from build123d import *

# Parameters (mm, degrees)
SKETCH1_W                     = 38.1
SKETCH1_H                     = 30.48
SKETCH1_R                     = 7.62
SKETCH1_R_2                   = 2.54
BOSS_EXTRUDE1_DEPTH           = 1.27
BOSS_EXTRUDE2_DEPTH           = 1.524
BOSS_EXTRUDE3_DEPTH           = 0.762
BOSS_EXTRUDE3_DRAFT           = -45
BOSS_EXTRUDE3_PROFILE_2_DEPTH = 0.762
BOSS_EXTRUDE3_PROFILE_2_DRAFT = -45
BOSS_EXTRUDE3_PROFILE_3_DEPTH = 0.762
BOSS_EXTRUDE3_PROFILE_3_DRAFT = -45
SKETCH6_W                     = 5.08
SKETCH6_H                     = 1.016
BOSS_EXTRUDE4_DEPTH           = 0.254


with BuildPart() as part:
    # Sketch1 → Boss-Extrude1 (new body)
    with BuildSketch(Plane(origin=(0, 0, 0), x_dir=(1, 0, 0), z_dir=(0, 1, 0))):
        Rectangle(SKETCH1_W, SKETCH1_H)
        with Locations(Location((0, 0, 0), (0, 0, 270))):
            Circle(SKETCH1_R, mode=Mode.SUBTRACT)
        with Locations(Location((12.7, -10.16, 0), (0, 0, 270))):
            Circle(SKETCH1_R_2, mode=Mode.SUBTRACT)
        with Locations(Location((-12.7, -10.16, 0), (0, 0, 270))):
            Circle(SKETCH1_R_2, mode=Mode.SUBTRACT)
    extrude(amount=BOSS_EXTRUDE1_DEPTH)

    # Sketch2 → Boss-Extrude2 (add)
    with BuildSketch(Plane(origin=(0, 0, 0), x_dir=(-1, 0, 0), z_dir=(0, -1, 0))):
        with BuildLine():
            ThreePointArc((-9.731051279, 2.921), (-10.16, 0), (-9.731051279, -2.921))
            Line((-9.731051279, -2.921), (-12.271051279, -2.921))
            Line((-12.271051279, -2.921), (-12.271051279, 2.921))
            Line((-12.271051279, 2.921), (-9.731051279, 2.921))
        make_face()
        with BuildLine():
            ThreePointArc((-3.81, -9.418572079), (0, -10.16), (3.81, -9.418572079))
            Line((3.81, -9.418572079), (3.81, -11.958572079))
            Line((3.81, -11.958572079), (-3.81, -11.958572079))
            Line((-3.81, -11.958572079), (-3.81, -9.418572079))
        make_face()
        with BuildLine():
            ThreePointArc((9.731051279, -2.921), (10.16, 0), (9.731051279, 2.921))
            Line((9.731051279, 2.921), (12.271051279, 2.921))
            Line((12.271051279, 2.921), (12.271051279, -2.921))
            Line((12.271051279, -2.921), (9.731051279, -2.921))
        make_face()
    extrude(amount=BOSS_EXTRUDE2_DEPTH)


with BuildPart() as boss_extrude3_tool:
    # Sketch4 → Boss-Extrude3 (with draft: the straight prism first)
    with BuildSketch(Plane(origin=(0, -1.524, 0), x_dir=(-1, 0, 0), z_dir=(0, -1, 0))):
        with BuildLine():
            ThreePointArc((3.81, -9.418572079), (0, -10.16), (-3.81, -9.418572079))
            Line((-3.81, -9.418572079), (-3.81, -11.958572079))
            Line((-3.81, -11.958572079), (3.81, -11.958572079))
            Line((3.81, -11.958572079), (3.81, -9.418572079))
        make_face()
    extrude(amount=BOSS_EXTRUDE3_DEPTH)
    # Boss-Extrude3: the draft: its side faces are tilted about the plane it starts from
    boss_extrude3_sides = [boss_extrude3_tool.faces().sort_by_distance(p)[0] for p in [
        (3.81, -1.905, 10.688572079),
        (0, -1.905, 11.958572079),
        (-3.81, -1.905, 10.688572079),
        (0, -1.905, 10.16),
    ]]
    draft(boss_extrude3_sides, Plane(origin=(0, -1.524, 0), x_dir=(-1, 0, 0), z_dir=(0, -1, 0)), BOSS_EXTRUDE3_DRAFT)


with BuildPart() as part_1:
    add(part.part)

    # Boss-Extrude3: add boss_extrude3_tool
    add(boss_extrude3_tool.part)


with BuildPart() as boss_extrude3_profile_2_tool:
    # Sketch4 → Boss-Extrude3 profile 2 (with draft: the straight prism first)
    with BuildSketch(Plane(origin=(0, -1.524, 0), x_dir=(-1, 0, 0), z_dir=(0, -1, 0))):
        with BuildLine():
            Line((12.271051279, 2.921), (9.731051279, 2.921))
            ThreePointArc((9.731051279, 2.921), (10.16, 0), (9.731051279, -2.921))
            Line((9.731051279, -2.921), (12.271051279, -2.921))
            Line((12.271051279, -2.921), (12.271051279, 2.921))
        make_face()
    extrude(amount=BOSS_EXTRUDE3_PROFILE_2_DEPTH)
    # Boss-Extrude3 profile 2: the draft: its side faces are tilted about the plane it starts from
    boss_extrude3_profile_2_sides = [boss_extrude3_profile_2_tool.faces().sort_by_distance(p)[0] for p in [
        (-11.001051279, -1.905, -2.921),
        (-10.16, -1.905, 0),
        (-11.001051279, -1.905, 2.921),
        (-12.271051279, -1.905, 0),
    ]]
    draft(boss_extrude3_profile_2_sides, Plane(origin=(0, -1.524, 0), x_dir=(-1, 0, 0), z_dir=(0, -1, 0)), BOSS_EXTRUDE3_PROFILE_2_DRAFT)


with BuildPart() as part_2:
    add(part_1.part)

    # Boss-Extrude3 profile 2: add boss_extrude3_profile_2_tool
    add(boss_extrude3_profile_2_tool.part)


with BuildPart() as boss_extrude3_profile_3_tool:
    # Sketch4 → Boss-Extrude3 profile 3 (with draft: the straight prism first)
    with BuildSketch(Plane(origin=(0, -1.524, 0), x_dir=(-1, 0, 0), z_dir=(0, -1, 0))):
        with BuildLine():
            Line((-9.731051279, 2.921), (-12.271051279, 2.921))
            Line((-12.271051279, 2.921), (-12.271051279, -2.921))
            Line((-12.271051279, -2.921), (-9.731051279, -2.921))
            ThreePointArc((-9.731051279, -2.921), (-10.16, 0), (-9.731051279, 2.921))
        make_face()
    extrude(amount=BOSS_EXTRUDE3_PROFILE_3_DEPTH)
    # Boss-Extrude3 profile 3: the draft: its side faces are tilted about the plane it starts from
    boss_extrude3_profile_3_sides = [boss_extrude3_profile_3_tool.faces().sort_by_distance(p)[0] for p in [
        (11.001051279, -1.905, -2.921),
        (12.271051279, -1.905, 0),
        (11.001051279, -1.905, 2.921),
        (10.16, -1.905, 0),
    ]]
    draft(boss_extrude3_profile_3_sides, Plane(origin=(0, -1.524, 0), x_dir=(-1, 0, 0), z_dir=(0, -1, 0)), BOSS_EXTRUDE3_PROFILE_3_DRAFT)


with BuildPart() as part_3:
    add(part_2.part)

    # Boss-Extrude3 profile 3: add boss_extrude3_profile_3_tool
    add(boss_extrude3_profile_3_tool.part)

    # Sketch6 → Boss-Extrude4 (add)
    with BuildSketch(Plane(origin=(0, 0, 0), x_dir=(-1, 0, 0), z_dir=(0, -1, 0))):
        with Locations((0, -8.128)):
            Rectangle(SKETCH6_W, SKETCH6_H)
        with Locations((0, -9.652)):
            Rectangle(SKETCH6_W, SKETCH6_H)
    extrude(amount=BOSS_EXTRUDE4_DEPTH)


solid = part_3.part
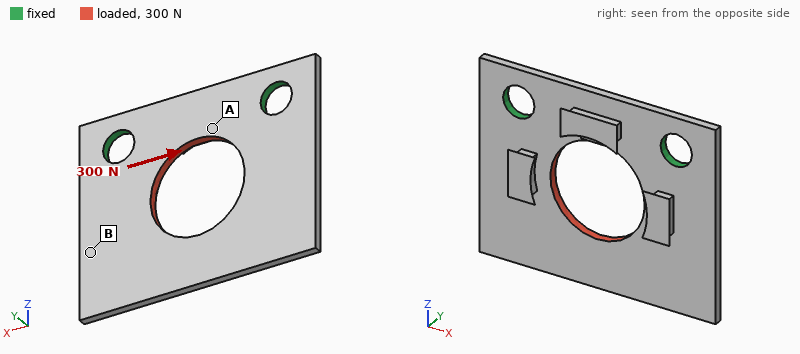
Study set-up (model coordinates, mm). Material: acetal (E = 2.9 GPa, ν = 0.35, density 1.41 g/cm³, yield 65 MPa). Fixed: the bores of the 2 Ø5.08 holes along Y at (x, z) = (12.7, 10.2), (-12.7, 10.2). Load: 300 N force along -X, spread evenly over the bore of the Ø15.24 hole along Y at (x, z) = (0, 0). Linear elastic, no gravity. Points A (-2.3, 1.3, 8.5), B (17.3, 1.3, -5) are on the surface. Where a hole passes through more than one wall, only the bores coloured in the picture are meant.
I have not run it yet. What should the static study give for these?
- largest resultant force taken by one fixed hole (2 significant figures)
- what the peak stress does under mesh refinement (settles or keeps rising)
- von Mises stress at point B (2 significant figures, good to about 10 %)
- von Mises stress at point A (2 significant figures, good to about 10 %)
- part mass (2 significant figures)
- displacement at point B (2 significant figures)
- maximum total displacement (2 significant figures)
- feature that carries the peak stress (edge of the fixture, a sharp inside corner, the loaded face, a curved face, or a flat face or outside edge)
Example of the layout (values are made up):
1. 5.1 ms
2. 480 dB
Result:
1. 170 N
2. keeps rising
3. 3.1 MPa
4. 13 MPa
5. 1.8 g
6. 0.17 mm
7. 0.24 mm
8. edge of the fixture
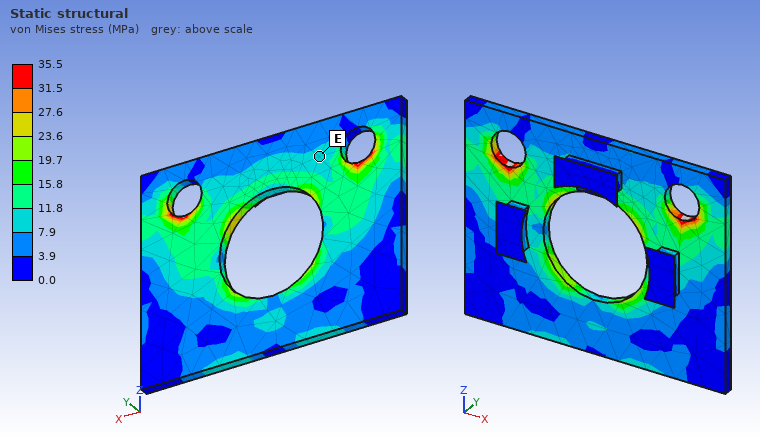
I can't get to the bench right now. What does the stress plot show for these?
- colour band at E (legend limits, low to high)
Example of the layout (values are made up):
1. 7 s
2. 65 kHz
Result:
1. 7.9 to 11.8 MPa
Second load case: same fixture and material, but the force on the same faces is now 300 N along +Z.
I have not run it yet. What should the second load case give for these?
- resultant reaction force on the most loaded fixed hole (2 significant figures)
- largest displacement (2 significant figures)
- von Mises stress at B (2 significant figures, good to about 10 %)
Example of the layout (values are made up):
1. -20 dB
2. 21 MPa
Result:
1. 150 N
2. 99 µm
3. 1.8 MPa
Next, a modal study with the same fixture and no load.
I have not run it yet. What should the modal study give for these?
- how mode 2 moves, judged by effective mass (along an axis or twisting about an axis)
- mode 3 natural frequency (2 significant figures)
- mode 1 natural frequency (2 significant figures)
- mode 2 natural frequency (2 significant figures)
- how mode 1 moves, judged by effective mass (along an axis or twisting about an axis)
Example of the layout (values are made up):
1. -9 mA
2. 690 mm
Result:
1. twisting about Z
2. 1900 Hz
3. 480 Hz
4. 870 Hz
5. along Y
